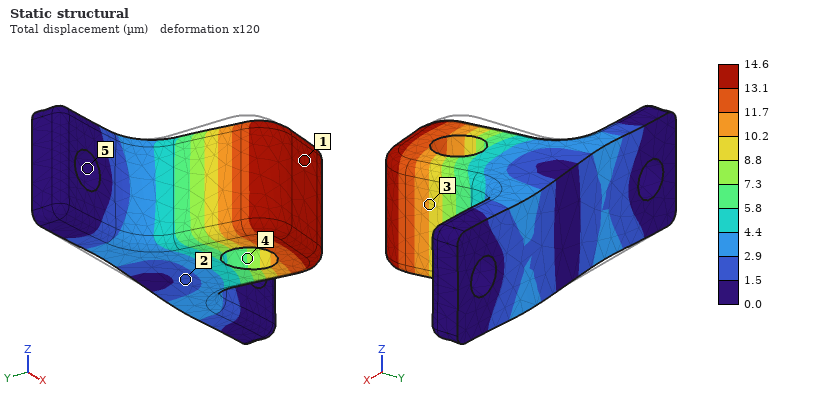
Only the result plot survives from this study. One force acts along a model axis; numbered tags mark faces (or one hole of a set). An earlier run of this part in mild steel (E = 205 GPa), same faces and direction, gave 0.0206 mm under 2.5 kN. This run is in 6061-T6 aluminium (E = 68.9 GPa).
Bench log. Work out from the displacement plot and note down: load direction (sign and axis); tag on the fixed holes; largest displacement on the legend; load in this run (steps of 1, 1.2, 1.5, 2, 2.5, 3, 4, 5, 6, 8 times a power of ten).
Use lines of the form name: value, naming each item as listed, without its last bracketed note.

load direction: +X
tag on the fixed holes: 5
largest displacement on the legend: 14.6 µm
load in this run: 600 N
